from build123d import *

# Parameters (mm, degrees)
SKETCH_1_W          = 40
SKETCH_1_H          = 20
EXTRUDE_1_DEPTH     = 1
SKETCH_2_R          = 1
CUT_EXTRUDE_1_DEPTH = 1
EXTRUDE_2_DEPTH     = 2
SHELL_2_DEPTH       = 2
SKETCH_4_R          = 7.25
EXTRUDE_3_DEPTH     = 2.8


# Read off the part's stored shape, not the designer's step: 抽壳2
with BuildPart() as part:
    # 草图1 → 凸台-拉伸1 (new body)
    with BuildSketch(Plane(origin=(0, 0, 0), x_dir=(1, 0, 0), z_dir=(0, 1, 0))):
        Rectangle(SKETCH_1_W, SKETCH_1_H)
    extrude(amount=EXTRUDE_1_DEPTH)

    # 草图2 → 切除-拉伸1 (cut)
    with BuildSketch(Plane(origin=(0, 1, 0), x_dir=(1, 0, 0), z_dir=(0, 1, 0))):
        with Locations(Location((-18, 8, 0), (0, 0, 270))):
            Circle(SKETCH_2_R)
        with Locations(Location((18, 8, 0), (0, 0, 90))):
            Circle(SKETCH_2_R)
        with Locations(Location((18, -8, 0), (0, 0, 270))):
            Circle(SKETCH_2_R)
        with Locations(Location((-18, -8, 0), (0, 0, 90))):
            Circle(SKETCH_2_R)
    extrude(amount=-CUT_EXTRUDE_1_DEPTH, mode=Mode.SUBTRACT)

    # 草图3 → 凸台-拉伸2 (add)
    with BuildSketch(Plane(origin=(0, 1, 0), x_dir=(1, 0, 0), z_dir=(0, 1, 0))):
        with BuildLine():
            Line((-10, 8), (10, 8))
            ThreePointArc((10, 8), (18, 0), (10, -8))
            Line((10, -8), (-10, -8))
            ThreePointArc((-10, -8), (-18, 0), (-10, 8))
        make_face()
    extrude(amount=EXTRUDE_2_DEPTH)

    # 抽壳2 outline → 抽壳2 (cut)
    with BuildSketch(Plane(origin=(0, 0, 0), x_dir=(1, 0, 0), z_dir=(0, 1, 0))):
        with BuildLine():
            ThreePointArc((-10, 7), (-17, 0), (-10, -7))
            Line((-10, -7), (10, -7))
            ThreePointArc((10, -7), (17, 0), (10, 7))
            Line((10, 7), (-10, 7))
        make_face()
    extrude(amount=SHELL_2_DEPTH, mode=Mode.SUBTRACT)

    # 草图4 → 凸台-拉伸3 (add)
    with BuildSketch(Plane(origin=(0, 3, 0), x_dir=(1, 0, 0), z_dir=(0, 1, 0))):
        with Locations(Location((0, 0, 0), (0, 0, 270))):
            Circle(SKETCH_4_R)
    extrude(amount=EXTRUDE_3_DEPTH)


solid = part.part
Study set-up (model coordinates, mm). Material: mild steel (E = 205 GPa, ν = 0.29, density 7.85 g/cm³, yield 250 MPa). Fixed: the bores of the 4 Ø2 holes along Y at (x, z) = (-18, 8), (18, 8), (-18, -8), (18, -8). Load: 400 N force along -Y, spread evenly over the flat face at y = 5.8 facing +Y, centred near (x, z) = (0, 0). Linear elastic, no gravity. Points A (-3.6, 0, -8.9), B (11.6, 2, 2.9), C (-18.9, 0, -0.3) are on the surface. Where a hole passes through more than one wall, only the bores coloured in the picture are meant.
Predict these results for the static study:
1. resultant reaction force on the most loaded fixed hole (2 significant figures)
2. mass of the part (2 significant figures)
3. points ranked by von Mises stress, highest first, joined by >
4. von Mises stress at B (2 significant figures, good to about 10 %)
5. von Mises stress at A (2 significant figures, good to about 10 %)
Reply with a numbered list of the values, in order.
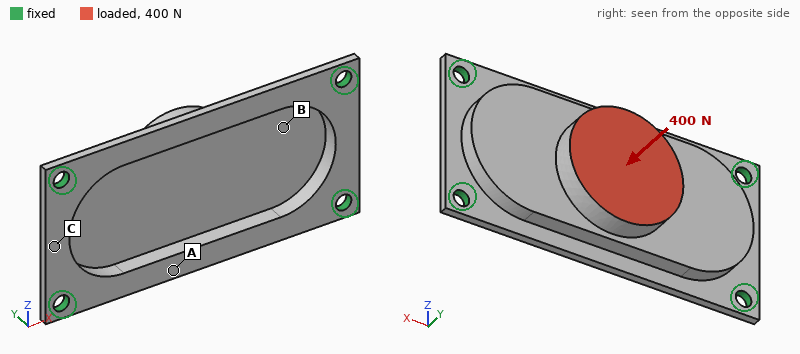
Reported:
1. 300 N
2. 11 g
3. A > B > C
4. 47 MPa
5. 65 MPa
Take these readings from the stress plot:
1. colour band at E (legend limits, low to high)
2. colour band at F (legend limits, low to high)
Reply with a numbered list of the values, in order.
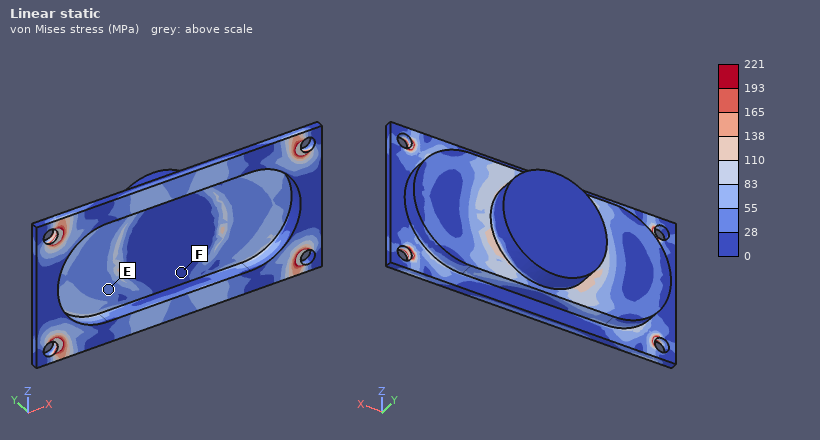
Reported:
1. 28 to 55 MPa
2. 0 to 28 MPa
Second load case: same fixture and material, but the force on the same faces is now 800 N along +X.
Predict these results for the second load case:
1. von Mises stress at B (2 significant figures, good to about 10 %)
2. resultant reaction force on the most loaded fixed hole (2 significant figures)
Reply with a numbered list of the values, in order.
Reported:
1. 33 MPa
2. 210 N
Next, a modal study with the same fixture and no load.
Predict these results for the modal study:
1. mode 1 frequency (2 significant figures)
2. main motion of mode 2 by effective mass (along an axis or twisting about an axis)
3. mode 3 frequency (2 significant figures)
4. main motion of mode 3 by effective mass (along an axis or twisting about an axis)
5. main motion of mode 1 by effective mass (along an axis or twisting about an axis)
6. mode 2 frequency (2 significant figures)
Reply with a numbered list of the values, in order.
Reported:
1. 7100 Hz
2. twisting about X
3. 17 kHz
4. twisting about Z
5. along Y
6. 8900 Hz
